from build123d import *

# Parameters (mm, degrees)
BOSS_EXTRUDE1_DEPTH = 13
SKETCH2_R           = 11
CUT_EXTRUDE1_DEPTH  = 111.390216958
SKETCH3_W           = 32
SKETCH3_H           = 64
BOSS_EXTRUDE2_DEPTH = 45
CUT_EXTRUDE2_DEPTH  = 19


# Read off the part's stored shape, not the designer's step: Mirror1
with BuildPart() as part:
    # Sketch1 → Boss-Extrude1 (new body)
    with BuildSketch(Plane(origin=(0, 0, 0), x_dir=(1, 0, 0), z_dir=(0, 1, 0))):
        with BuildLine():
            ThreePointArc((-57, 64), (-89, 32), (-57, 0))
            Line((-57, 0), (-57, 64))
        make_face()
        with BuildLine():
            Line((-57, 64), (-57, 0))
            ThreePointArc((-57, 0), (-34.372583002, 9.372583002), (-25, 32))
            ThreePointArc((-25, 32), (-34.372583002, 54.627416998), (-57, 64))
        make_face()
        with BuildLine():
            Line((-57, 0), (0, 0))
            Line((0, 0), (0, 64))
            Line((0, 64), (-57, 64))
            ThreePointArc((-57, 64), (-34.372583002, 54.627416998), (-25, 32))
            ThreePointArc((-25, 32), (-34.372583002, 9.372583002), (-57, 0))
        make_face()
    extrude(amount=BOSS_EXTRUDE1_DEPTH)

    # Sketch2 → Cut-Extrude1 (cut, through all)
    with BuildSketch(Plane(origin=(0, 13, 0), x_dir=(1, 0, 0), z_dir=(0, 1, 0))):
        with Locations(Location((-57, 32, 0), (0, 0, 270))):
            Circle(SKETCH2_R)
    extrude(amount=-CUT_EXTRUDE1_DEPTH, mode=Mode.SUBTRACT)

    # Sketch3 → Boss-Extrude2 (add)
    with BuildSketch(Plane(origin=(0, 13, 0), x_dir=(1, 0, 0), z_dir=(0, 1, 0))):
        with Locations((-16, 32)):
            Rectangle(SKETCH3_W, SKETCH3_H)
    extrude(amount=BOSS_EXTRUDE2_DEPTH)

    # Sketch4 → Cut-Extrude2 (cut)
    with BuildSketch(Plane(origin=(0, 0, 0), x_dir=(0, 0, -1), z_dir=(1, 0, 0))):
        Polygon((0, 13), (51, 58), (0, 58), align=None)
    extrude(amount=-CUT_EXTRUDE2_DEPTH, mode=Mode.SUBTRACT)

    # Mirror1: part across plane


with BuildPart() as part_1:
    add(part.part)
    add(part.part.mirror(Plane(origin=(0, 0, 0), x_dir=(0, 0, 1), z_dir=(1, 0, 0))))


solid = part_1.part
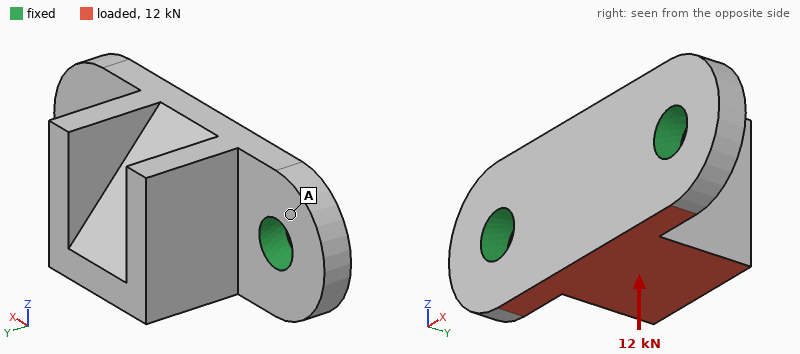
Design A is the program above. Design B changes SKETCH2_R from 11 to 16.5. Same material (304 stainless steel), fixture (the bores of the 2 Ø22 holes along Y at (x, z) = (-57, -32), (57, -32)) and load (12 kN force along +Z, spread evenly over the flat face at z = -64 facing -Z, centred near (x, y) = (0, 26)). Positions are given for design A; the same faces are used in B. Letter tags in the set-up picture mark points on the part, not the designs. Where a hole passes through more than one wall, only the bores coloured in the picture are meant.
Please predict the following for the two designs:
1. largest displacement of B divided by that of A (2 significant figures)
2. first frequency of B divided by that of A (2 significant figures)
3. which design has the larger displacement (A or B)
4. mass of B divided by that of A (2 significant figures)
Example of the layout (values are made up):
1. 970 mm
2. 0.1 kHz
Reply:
1. 0.62
2. 1.3
3. A
4. 0.95
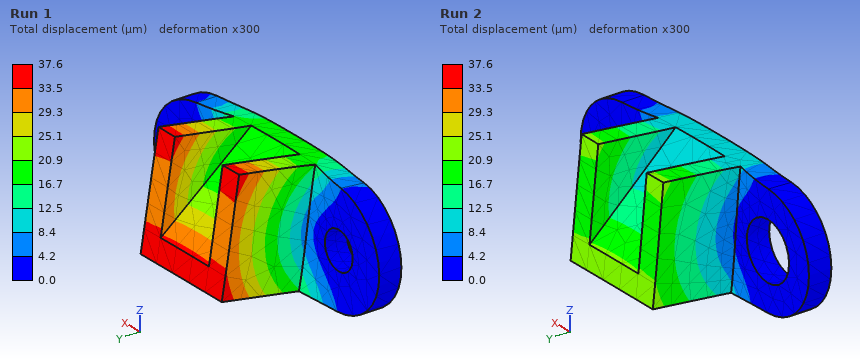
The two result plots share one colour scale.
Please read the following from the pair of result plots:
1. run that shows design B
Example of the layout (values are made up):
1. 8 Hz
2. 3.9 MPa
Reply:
1. Run 2
